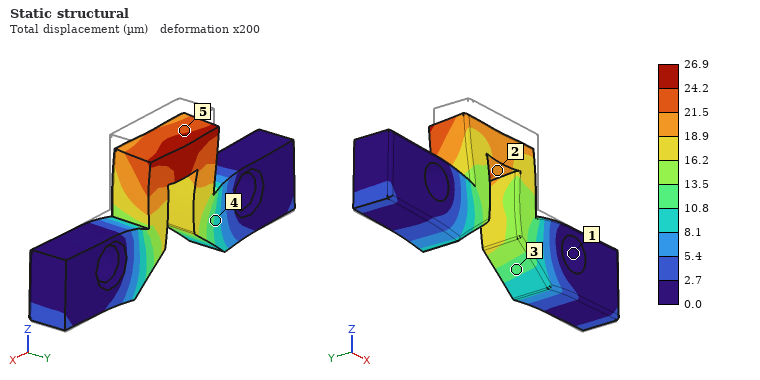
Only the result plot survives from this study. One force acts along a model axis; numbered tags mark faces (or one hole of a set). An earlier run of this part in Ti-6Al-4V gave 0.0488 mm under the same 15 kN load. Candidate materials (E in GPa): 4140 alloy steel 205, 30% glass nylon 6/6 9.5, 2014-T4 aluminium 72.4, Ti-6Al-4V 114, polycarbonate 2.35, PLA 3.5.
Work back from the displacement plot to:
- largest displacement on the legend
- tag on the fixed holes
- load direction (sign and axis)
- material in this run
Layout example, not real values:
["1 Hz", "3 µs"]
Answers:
["26.9 µm", "1", "-Z", "4140 alloy steel"]
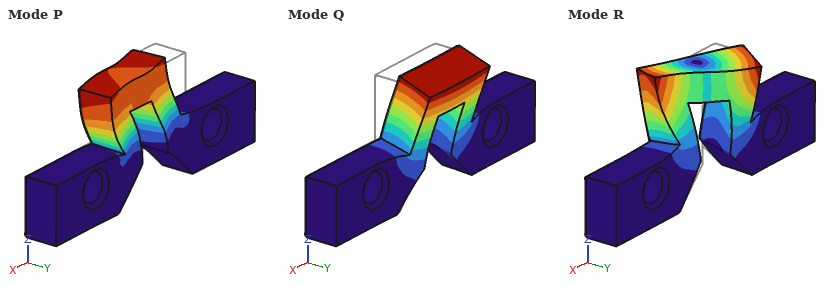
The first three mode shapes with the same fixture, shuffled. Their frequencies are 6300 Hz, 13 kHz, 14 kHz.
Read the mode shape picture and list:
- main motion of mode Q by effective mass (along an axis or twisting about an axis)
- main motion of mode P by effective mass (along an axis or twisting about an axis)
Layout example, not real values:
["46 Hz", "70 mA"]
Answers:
["along Y", "along X"]
